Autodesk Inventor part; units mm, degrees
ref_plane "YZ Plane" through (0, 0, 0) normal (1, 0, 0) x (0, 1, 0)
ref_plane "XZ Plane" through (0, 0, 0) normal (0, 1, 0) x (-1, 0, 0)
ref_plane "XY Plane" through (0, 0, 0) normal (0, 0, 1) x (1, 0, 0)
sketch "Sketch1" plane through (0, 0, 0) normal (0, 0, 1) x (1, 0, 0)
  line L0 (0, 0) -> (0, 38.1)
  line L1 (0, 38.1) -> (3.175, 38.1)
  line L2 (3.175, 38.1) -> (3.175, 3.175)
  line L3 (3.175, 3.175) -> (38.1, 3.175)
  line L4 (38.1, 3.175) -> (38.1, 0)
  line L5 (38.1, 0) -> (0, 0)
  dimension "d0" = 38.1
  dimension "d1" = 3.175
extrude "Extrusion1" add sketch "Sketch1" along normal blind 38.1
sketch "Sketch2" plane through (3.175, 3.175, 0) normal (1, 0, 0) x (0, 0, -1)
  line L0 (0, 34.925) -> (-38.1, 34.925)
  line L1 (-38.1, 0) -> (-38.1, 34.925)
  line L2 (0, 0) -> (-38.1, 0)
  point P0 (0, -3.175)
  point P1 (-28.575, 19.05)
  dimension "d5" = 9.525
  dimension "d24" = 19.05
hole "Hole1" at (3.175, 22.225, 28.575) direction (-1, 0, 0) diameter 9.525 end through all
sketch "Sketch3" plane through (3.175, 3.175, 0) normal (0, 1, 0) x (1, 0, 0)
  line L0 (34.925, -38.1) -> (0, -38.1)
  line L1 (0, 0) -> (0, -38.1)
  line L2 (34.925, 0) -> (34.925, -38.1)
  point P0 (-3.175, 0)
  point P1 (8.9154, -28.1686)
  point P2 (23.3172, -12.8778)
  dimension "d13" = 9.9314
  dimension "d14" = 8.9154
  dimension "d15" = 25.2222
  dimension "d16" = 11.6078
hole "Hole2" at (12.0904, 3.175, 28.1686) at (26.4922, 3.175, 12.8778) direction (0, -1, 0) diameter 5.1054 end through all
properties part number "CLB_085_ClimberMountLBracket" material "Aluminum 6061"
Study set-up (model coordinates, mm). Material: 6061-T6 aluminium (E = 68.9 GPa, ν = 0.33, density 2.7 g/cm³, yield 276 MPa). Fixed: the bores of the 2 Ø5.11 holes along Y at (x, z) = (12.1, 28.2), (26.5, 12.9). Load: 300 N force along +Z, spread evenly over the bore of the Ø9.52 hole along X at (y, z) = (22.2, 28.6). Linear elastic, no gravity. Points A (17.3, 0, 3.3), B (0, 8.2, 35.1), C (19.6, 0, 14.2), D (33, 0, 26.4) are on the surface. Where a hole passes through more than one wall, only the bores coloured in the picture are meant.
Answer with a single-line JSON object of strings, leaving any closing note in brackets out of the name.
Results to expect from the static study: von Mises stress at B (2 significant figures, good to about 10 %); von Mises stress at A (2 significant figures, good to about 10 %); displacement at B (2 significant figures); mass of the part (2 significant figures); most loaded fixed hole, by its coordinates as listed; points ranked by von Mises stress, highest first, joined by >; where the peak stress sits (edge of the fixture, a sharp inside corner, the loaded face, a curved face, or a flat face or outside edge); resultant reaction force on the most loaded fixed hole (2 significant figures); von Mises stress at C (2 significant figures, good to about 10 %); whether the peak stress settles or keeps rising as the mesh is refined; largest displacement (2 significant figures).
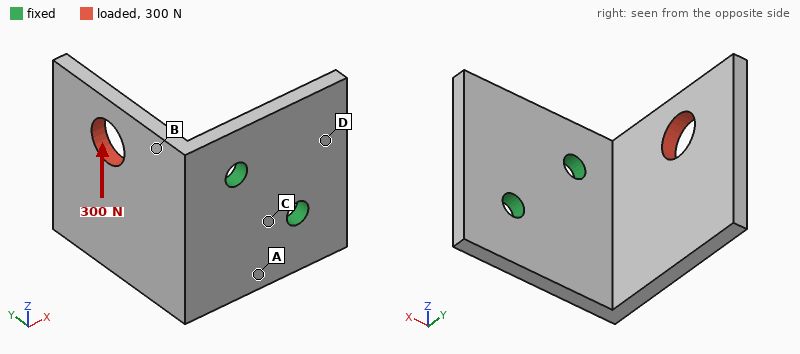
{"von Mises stress at B": "20 MPa", "von Mises stress at A": "34 MPa", "displacement at B": "0.043 mm", "mass of the part": "23 g", "most loaded fixed hole, by its coordinates as listed": "(12.1, 28.2)", "points ranked by von Mises stress, highest first, joined by >": "C > A > B > D", "where the peak stress sits": "edge of the fixture", "resultant reaction force on the most loaded fixed hole": "360 N", "von Mises stress at C": "42 MPa", "whether the peak stress settles or keeps rising as the mesh is refined": "keeps rising", "largest displacement": "0.24 mm"}
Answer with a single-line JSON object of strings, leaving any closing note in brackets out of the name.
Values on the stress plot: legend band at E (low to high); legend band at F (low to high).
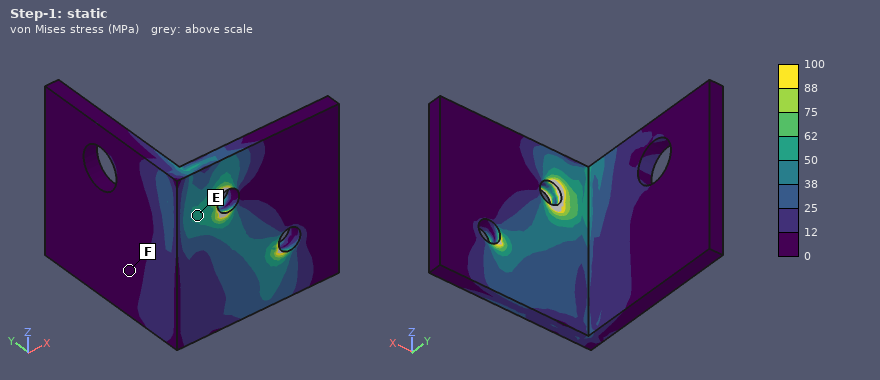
{"legend band at E": "50 to 62 MPa", "legend band at F": "0 to 12 MPa"}
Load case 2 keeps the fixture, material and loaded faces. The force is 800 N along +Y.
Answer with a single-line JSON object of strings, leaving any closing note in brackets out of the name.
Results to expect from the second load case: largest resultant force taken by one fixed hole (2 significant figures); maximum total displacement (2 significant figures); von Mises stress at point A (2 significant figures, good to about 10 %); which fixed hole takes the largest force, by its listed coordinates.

{"largest resultant force taken by one fixed hole": "880 N", "maximum total displacement": "0.26 mm", "von Mises stress at point A": "19 MPa", "which fixed hole takes the largest force, by its listed coordinates": "(12.1, 28.2)"}
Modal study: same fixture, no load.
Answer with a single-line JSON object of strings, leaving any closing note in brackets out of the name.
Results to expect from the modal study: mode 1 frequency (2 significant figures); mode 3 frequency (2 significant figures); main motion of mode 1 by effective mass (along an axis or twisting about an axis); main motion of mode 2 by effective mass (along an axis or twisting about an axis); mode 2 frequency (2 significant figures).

{"mode 1 frequency": "1300 Hz", "mode 3 frequency": "4100 Hz", "main motion of mode 1 by effective mass": "along X", "main motion of mode 2 by effective mass": "along Z", "mode 2 frequency": "2200 Hz"}
